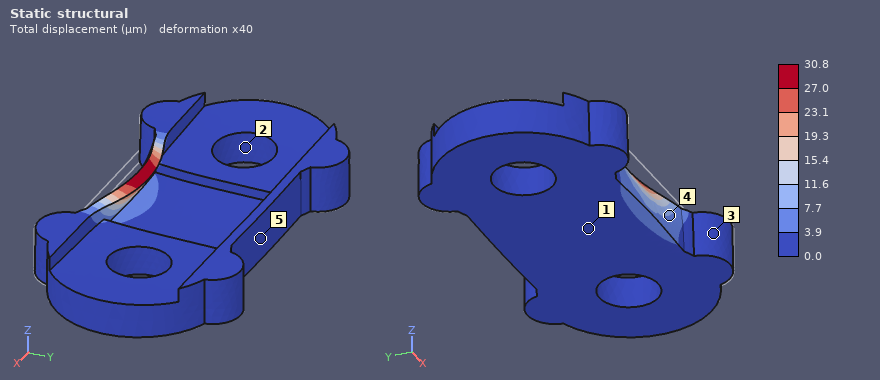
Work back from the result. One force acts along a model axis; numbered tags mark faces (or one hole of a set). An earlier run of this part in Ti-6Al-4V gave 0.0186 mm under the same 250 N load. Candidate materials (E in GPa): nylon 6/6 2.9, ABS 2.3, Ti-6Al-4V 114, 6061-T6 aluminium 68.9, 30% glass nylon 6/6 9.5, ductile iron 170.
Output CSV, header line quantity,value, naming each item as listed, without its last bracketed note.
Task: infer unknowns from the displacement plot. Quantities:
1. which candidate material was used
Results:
quantity,value
which candidate material was used,6061-T6 aluminium
